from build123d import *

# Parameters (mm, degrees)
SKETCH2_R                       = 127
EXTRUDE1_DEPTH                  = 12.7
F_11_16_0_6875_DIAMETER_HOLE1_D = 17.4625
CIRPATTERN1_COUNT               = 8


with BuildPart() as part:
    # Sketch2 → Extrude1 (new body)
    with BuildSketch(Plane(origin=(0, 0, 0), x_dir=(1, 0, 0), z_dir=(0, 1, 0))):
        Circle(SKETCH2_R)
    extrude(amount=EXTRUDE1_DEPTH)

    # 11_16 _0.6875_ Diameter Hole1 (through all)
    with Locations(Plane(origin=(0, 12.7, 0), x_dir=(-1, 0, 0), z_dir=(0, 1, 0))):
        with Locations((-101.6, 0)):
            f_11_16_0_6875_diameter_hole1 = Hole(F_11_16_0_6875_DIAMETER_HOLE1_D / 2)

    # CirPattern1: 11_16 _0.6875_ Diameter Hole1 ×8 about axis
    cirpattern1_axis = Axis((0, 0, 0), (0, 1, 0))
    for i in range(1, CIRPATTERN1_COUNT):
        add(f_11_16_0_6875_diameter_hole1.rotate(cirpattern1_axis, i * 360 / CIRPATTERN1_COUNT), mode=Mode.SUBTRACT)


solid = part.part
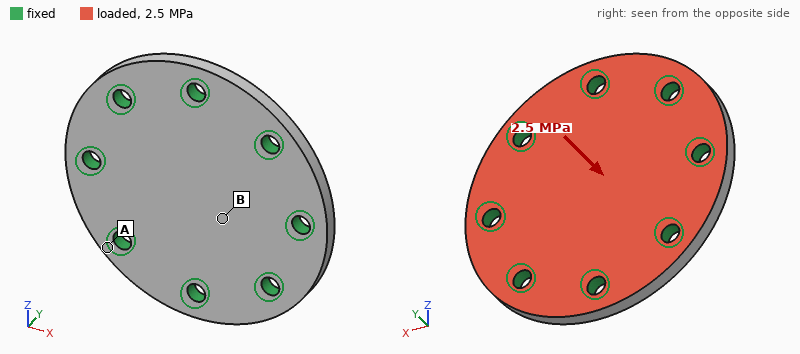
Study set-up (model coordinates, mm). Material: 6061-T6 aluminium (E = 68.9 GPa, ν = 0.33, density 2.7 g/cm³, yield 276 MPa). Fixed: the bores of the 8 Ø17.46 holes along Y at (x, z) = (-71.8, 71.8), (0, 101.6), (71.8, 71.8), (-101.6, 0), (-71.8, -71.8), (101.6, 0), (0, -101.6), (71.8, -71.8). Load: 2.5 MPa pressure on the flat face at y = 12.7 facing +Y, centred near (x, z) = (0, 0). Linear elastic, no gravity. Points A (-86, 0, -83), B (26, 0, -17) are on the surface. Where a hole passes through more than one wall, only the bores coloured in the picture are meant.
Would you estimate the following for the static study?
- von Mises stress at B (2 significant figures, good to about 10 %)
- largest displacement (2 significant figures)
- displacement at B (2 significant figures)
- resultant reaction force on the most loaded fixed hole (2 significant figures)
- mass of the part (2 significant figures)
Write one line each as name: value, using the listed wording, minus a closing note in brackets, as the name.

von Mises stress at B: 61 MPa
largest displacement: 0.32 mm
displacement at B: 0.26 mm
resultant reaction force on the most loaded fixed hole: 15 kN
mass of the part: 1.7 kg
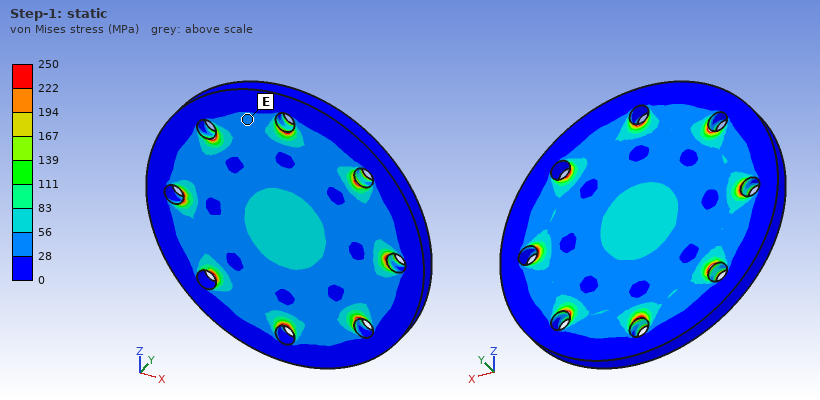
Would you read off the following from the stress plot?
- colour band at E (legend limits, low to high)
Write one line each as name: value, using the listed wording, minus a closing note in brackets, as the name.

colour band at E: 28 to 56 MPa
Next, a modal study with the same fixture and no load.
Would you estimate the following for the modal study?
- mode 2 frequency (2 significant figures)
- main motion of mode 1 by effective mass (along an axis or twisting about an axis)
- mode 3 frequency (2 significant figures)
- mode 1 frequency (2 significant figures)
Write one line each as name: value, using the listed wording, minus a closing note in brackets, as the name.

mode 2 frequency: 5900 Hz
main motion of mode 1 by effective mass: along Y
mode 3 frequency: 5900 Hz
mode 1 frequency: 3000 Hz
